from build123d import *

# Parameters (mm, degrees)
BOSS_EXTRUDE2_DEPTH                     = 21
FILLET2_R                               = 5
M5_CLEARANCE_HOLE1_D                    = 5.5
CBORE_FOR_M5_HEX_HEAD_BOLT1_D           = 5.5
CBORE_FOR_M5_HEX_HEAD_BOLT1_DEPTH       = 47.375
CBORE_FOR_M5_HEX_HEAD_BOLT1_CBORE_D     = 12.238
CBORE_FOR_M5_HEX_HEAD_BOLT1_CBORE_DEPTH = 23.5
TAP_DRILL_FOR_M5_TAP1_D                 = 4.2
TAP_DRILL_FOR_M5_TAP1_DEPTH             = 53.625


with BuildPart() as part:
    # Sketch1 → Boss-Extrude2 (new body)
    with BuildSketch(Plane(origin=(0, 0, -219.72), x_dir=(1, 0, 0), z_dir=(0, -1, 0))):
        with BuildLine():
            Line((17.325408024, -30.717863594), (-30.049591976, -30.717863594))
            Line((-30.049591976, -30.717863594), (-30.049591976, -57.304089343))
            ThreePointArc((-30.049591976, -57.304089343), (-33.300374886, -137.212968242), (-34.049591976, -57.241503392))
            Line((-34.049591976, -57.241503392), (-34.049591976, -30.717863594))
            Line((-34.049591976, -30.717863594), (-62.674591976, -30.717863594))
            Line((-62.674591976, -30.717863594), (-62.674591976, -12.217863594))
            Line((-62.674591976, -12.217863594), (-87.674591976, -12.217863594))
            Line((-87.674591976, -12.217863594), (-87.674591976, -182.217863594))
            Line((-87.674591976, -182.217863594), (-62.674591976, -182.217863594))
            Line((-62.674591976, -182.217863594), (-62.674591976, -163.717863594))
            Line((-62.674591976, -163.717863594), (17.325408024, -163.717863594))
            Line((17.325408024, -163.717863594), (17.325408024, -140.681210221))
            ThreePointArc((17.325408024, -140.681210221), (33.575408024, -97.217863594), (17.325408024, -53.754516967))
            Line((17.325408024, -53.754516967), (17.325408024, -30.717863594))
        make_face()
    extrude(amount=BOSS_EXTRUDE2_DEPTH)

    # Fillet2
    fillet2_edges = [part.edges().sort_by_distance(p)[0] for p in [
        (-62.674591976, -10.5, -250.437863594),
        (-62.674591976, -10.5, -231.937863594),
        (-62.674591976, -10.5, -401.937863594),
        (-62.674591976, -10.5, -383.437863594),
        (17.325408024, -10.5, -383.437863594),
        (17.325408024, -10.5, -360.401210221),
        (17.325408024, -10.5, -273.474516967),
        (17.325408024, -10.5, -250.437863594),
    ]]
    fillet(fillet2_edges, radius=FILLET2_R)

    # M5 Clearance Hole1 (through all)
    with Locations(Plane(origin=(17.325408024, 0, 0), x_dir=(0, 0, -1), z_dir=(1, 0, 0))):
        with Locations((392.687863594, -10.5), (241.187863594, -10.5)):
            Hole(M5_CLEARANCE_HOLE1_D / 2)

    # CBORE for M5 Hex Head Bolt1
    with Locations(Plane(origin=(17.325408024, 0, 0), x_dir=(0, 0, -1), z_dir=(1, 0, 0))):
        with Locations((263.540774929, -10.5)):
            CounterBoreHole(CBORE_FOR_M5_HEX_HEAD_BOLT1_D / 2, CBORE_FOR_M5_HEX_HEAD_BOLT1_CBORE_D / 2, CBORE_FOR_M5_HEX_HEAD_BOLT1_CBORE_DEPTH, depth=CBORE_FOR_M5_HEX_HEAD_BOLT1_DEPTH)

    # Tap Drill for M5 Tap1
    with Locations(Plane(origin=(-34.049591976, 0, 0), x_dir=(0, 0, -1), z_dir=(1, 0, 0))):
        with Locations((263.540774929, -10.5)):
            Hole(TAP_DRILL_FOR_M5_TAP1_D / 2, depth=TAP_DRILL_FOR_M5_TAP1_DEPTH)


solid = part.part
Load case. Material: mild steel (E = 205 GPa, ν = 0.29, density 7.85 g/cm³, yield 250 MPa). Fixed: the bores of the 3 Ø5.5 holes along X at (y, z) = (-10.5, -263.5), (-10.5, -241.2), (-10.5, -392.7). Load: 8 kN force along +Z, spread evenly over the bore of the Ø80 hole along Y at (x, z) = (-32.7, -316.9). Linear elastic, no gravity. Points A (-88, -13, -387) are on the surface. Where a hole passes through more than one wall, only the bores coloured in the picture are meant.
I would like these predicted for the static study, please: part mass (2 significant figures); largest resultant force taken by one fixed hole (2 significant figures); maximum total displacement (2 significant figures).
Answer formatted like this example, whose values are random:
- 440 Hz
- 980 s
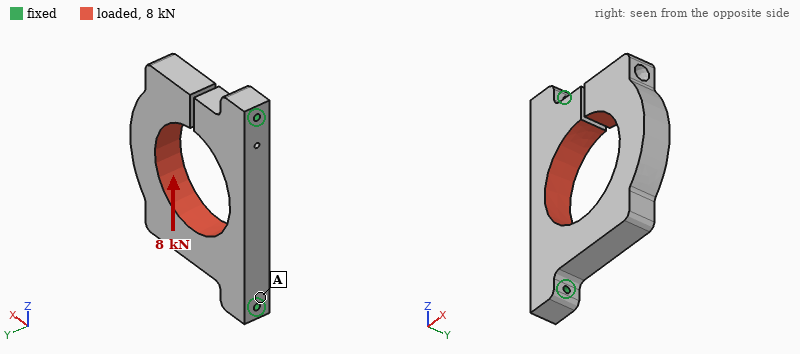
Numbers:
- 1.7 kg
- 3.2 kN
- 5.2 µm
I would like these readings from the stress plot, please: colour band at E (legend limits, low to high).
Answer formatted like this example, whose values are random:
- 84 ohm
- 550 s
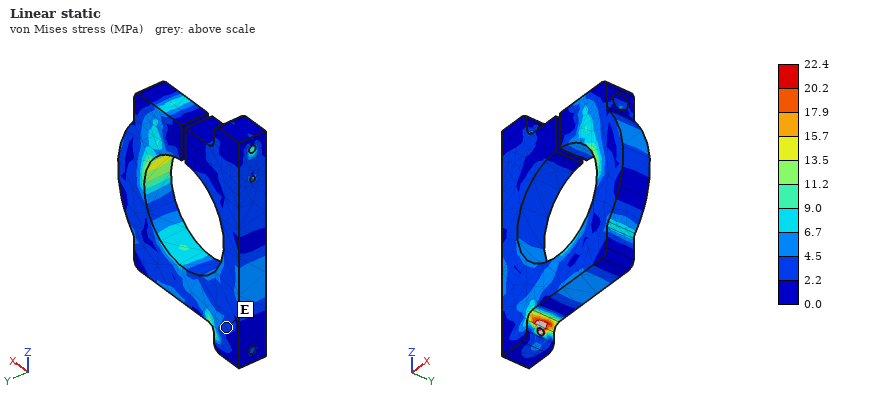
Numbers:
- 2.2 to 4.5 MPa
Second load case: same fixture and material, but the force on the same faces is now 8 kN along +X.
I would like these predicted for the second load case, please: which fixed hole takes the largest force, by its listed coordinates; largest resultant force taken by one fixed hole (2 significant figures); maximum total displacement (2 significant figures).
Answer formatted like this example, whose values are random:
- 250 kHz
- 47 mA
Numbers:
- (-10.5, -392.7)
- 4.2 kN
- 12 µm
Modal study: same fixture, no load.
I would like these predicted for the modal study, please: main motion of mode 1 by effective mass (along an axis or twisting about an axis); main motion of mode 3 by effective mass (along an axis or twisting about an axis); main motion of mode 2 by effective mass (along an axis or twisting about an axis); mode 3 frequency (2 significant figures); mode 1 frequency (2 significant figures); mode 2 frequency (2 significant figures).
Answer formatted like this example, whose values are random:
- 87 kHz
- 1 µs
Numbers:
- along Y
- along X
- along Y
- 4400 Hz
- 1600 Hz
- 3400 Hz
